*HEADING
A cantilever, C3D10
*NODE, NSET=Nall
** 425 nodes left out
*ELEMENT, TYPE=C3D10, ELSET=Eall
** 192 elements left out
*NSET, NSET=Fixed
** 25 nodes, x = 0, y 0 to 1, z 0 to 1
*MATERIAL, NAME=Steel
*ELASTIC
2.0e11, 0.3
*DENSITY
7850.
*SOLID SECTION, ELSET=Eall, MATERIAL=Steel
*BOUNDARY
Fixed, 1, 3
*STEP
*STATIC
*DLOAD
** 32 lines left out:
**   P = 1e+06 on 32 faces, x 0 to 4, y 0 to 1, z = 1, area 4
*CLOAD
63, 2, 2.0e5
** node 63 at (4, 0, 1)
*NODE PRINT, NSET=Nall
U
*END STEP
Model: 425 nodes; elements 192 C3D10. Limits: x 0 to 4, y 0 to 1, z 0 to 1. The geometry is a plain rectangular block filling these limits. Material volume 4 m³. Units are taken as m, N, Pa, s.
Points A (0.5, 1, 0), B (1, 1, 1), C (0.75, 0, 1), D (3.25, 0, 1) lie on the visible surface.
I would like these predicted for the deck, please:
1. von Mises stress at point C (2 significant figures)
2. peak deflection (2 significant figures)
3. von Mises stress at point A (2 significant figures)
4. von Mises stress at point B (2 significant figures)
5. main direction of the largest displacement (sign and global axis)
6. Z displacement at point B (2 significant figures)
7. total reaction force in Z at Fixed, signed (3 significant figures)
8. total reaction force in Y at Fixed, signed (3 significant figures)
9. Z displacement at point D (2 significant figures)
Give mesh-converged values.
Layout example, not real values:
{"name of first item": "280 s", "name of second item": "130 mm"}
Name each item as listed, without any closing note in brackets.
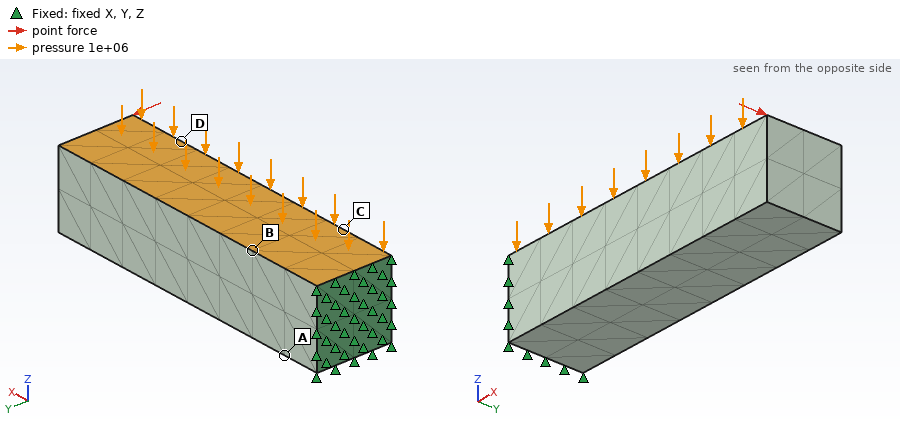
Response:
{"von Mises stress at point C": "3.5e+07 Pa", "peak deflection": "0.0021 m", "von Mises stress at point A": "4.0e+07 Pa", "von Mises stress at point B": "2.4e+07 Pa", "main direction of the largest displacement": "-Z", "Z displacement at point B": "-2.5e-04 m", "total reaction force in Z at Fixed, signed": "4.00e+06 N", "total reaction force in Y at Fixed, signed": "-2.00e+05 N", "Z displacement at point D": "-0.0015 m"}
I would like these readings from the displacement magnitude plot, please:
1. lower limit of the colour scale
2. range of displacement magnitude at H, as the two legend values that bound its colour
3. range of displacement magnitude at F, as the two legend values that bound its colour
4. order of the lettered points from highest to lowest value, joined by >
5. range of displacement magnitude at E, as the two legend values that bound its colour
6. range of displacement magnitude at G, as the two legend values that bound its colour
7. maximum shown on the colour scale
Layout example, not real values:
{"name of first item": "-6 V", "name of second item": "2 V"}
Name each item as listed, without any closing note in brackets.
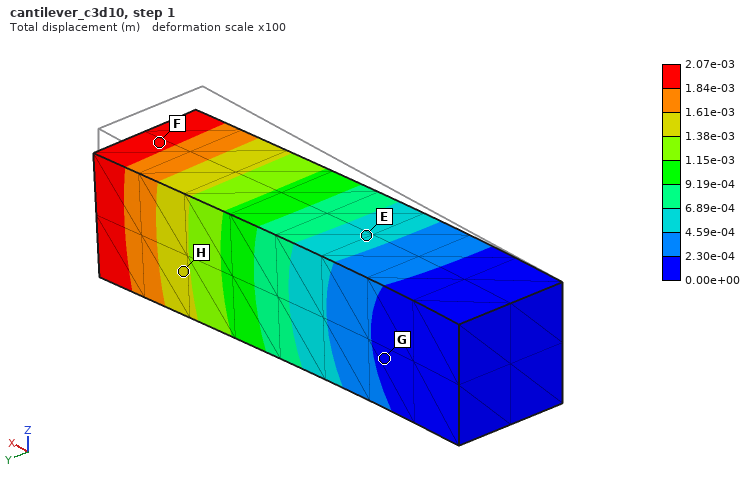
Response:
{"lower limit of the colour scale": "0.00e+00 m", "range of displacement magnitude at H, as the two legend values that bound its colour": "1.38e-03 to 1.61e-03 m", "range of displacement magnitude at F, as the two legend values that bound its colour": "1.84e-03 to 2.07e-03 m", "order of the lettered points from highest to lowest value, joined by >": "F > H > E > G", "range of displacement magnitude at E, as the two legend values that bound its colour": "4.59e-04 to 6.89e-04 m", "range of displacement magnitude at G, as the two legend values that bound its colour": "0.00e+00 to 2.30e-04 m", "maximum shown on the colour scale": "2.07e-03 m"}
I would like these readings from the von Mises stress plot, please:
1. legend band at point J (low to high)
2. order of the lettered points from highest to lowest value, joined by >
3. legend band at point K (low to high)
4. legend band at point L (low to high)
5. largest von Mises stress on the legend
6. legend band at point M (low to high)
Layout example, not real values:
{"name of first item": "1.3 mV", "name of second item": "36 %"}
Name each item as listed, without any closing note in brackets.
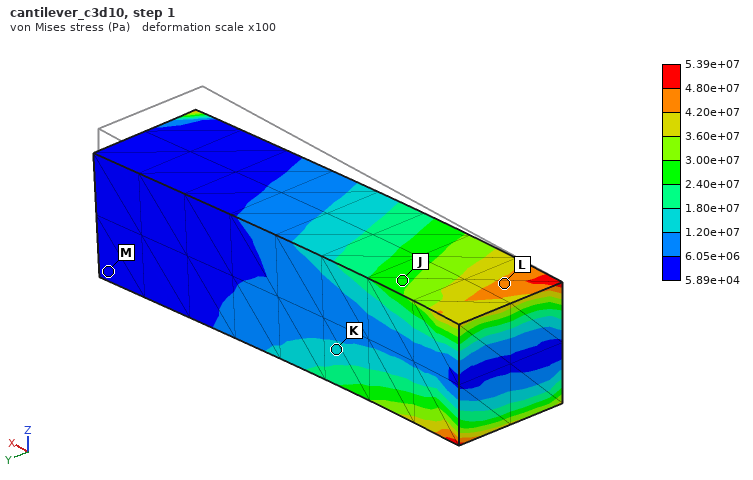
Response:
{"legend band at point J": "2.40e+07 to 3.00e+07 Pa", "order of the lettered points from highest to lowest value, joined by >": "L > J > K > M", "legend band at point K": "1.20e+07 to 1.80e+07 Pa", "legend band at point L": "4.20e+07 to 4.80e+07 Pa", "largest von Mises stress on the legend": "5.39e+07 Pa", "legend band at point M": "5.89e+04 to 6.05e+06 Pa"}
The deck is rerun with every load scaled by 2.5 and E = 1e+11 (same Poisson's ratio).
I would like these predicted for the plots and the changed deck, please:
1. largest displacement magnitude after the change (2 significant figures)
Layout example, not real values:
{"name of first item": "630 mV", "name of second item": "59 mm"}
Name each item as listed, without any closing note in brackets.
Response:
{"largest displacement magnitude after the change": "0.010 m"}
